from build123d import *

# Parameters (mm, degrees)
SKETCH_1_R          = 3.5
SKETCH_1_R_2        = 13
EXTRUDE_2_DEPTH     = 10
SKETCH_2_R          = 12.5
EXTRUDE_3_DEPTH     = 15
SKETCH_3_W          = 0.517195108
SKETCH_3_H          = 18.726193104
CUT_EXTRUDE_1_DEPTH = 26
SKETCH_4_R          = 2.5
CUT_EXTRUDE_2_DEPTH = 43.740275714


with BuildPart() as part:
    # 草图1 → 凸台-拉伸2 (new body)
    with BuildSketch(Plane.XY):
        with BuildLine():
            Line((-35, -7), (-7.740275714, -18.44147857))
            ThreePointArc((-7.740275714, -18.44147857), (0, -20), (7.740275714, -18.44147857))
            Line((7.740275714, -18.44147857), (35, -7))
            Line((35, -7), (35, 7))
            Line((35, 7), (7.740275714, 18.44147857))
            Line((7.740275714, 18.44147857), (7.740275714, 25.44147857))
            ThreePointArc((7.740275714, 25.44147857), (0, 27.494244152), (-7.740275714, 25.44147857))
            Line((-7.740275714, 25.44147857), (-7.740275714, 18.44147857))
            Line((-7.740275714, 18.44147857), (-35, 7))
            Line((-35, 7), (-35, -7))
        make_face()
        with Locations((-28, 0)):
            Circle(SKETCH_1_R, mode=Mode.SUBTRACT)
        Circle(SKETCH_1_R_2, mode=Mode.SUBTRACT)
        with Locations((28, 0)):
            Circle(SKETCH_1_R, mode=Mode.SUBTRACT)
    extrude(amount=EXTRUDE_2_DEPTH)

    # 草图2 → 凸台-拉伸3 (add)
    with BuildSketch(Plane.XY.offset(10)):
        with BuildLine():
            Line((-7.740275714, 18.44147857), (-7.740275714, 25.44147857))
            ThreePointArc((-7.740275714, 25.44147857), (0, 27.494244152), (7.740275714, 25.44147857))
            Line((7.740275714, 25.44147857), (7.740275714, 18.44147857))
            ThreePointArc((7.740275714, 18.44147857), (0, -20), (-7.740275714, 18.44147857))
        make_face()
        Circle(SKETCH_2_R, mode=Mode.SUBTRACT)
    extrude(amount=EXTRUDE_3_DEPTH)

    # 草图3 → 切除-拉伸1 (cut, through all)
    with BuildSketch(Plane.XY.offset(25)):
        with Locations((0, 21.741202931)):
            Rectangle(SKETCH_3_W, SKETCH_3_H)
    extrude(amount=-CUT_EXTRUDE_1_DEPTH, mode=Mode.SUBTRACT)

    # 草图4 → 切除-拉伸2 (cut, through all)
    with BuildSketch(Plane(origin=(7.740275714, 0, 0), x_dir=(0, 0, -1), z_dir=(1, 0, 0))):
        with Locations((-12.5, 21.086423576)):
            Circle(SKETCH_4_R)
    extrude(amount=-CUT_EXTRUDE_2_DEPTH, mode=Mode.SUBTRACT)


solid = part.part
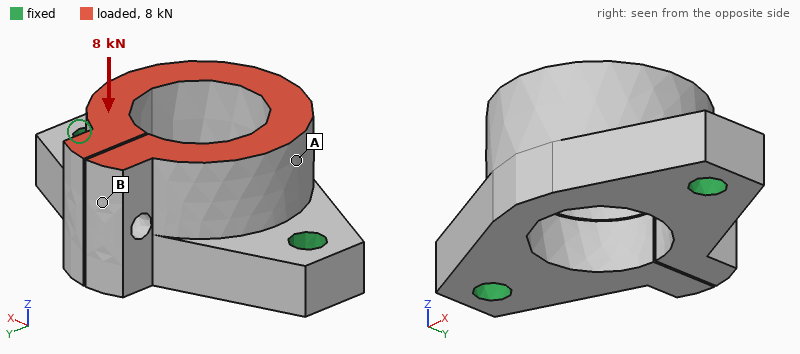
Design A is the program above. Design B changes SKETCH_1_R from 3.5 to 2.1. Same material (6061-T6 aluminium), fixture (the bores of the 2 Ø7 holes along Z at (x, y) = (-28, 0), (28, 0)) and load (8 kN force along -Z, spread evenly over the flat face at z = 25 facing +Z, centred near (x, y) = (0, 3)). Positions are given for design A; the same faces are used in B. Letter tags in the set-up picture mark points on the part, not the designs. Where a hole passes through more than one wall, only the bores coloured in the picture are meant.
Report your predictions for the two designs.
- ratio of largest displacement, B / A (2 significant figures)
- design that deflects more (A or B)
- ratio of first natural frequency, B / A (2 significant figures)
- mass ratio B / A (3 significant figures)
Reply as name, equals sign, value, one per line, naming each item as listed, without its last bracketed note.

ratio of largest displacement, B / A = 1.2
design that deflects more = B
ratio of first natural frequency, B / A = 0.89
mass ratio B / A = 1.02
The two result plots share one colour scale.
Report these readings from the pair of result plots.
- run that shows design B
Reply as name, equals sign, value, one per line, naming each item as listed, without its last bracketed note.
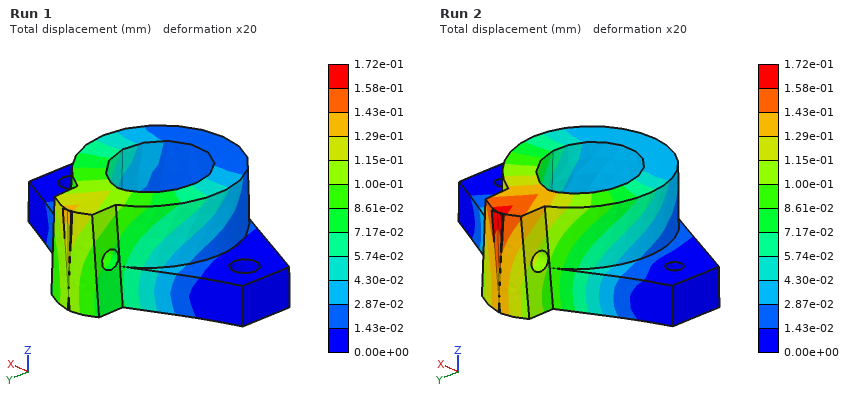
run that shows design B = Run 2
